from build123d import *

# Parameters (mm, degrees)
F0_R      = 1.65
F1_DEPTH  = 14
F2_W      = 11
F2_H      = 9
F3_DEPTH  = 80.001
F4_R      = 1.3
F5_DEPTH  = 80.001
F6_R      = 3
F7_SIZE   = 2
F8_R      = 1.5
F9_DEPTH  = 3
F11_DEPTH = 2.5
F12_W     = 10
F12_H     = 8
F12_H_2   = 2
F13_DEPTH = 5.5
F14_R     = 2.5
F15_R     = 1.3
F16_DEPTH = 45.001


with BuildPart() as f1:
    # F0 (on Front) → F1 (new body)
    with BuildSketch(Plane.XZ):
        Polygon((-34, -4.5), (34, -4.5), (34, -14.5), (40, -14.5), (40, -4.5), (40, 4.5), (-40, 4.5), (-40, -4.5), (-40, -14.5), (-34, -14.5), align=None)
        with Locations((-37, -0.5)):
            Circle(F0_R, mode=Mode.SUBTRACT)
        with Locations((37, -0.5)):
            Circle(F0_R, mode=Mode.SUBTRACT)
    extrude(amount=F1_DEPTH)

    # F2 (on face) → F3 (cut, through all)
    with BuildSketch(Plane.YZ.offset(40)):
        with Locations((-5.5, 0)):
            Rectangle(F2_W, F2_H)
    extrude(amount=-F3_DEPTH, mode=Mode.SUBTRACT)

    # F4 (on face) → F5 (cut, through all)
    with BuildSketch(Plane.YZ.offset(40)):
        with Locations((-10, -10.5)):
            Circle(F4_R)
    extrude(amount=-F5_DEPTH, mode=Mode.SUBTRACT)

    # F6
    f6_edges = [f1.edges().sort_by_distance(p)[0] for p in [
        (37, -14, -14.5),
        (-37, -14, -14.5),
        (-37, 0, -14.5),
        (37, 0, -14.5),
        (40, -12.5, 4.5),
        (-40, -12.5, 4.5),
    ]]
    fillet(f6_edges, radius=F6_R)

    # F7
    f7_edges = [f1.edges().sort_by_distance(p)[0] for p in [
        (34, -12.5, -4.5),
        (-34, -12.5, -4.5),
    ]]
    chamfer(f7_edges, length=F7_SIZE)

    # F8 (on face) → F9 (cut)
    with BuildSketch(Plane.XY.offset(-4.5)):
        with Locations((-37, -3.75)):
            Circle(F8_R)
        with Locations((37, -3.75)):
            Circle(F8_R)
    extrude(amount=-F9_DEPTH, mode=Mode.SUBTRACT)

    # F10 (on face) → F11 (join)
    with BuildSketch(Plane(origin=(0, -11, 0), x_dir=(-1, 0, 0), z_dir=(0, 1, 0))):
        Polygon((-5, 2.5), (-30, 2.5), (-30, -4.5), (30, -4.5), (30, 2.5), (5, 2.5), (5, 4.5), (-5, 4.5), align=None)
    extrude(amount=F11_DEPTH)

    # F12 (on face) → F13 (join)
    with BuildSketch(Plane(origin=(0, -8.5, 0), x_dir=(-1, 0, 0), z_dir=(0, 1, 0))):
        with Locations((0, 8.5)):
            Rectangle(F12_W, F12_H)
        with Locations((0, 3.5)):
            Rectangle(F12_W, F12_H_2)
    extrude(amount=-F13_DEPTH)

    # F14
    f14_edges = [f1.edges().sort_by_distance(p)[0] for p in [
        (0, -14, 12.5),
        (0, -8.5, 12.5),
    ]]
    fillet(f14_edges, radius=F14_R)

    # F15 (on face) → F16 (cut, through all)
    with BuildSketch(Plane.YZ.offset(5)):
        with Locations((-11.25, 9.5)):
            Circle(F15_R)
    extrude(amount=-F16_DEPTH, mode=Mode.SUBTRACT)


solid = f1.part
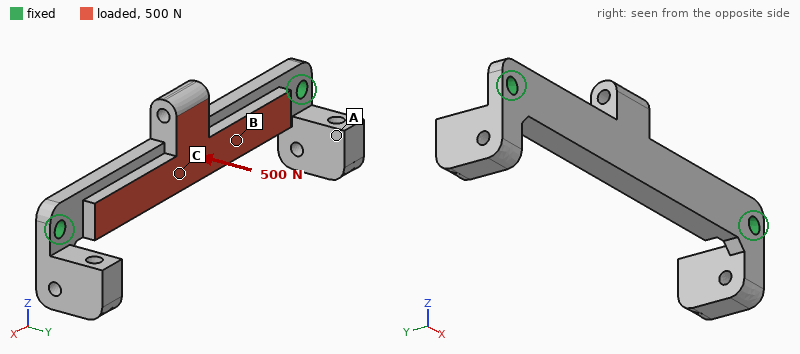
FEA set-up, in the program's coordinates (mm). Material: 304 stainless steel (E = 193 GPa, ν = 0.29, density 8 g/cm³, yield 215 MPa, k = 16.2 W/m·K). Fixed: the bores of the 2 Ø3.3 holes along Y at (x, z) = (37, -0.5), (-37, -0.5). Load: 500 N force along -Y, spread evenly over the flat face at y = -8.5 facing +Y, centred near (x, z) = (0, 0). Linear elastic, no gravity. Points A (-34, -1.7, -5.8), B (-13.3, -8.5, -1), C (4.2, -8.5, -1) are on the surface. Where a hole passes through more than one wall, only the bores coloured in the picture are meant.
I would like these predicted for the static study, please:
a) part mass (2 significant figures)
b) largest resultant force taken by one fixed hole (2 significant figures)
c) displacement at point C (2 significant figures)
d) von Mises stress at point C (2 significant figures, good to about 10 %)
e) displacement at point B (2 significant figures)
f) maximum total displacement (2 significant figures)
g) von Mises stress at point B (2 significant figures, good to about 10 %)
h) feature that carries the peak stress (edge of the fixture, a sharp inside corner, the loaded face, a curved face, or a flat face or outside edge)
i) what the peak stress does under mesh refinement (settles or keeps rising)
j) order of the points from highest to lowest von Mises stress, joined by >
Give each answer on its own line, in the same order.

41 g
550 N
54 µm
80 MPa
44 µm
63 µm
66 MPa
edge of the fixture
keeps rising
C > B > A
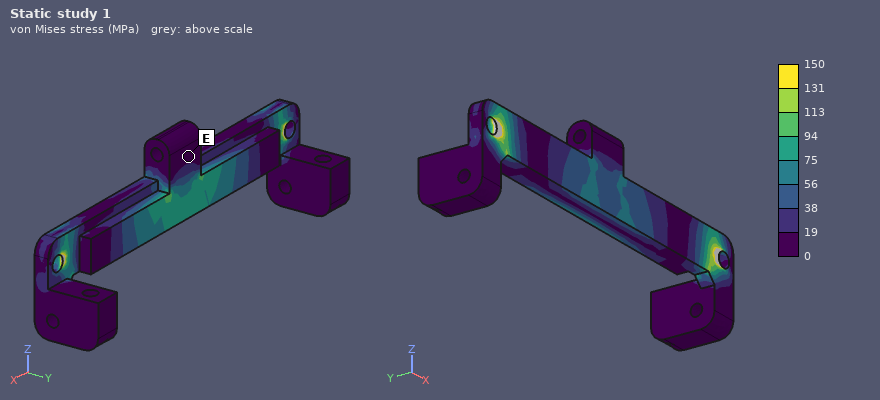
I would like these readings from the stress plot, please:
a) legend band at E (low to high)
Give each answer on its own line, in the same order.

0 to 19 MPa
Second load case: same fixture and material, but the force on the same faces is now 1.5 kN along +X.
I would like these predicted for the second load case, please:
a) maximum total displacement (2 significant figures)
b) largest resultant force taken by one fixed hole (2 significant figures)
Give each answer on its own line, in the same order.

5.0 µm
760 N
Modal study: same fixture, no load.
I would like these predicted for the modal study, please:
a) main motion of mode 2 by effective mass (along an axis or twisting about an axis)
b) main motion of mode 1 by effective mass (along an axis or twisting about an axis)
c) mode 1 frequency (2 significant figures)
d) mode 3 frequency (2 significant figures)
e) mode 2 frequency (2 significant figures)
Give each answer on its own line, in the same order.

along Z
along Y
3300 Hz
5700 Hz
5300 Hz
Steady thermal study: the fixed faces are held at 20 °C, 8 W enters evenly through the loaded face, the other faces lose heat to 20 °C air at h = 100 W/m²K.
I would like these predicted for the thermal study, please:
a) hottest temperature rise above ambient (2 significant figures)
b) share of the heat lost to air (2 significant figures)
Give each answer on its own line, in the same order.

46 K
74 %
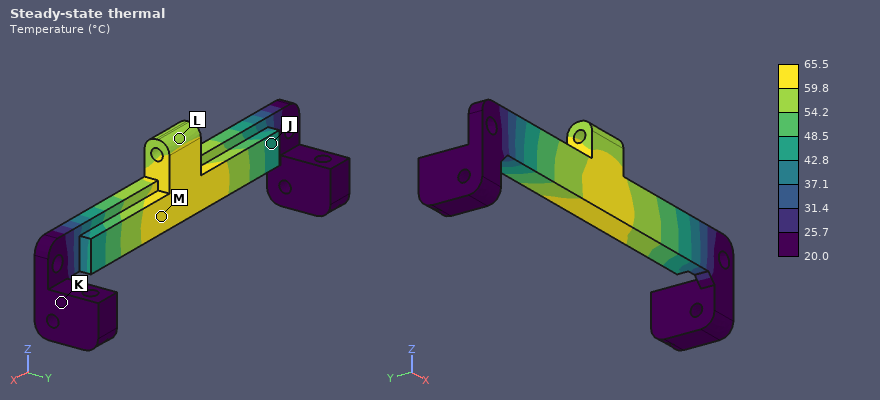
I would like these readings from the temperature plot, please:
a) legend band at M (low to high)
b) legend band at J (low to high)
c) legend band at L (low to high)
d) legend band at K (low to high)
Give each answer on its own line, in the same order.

59.8 to 65.5 °C
42.8 to 48.5 °C
54.2 to 59.8 °C
20.0 to 25.7 °C
